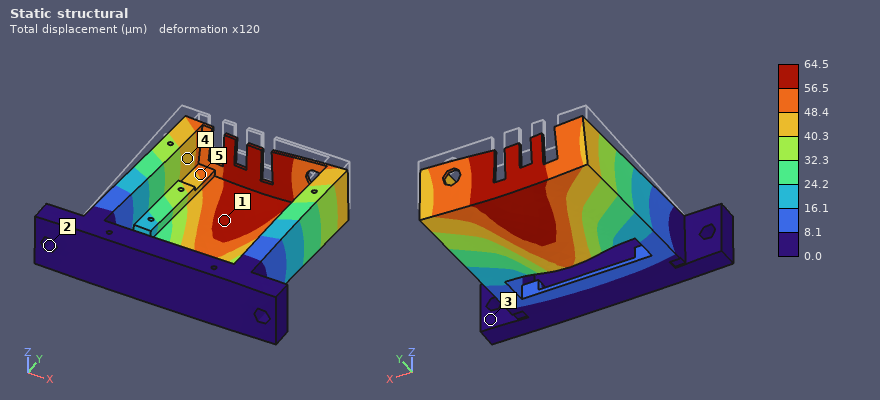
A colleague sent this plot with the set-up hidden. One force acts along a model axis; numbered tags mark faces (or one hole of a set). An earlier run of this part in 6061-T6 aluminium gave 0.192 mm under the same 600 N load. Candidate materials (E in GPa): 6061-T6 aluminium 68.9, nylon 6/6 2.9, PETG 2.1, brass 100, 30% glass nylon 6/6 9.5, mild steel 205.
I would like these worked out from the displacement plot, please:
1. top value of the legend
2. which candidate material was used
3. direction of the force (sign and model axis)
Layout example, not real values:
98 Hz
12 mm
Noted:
64.5 µm
mild steel
-Z
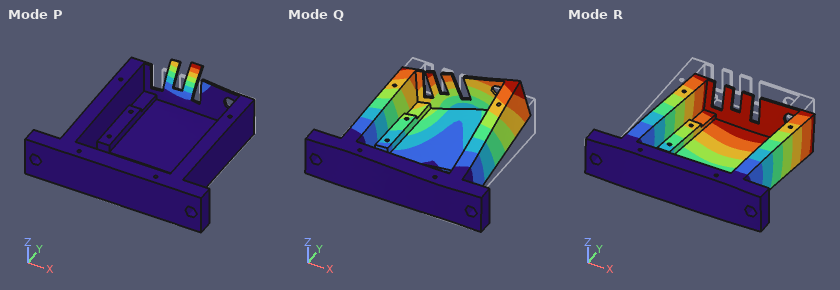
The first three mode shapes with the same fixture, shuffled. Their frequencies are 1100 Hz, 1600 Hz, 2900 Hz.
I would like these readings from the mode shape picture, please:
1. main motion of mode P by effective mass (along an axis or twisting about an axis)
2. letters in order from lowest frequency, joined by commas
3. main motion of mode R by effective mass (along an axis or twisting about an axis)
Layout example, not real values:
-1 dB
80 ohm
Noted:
along X
R, Q, P
along Z
